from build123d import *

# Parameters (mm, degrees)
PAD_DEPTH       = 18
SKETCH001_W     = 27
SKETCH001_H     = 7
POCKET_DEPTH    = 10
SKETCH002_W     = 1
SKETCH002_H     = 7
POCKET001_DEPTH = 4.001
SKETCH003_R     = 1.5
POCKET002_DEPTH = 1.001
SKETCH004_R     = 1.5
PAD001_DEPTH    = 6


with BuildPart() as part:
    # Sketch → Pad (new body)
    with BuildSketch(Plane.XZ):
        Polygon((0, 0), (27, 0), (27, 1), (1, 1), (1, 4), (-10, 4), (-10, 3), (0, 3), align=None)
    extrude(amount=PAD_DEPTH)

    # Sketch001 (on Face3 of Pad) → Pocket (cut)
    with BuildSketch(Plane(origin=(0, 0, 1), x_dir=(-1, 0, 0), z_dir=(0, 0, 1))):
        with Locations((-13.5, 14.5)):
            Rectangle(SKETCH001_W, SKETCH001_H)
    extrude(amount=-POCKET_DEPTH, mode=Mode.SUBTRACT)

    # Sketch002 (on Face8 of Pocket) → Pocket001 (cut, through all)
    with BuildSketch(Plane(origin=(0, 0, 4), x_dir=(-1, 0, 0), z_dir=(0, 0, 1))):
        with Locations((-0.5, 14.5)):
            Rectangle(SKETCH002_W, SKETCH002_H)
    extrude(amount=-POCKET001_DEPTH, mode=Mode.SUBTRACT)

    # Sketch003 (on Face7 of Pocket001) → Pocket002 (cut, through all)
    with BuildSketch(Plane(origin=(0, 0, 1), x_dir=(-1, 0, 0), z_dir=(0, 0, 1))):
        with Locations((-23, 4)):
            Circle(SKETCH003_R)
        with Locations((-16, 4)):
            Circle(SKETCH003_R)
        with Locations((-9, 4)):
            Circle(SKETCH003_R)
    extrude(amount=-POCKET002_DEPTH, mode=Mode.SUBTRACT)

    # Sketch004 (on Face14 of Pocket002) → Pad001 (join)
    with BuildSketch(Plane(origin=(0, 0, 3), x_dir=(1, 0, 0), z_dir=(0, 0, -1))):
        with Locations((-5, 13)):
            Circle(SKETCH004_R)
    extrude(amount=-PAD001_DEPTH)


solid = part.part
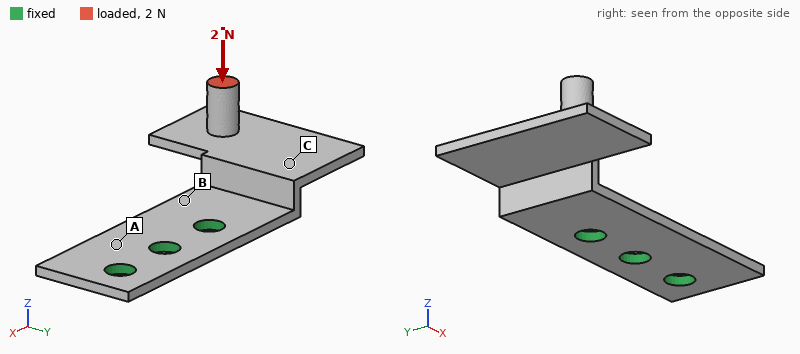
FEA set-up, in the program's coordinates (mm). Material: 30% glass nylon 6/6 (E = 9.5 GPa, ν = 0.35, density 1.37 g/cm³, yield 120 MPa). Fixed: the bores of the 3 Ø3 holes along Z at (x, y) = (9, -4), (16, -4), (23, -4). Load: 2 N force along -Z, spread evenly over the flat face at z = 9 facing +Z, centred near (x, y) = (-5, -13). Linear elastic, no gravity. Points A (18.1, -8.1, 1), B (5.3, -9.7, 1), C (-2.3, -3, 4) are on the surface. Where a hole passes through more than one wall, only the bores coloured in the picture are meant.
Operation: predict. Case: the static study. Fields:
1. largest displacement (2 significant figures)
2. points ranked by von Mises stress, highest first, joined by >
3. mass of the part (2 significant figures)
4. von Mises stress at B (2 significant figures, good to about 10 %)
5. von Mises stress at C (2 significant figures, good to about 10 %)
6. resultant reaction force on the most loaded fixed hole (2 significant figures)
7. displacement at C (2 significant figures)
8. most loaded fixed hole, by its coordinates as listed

0.49 mm
B > C > A
0.72 g
11 MPa
4.3 MPa
2.8 N
0.12 mm
(9, -4)
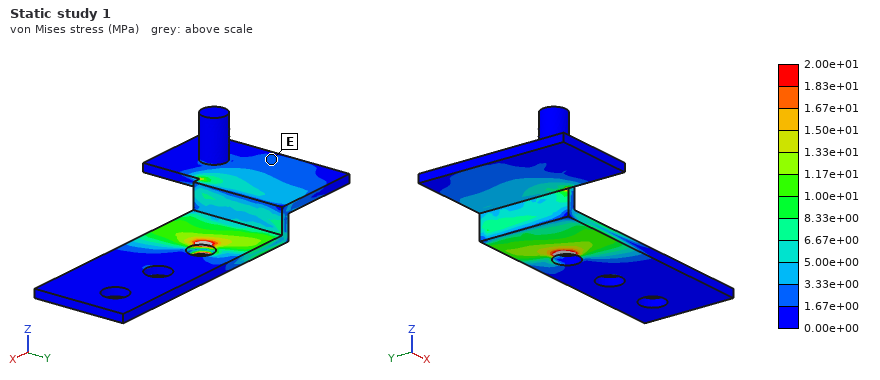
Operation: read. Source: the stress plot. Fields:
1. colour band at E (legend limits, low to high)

1.67e+00 to 3.33e+00 MPa
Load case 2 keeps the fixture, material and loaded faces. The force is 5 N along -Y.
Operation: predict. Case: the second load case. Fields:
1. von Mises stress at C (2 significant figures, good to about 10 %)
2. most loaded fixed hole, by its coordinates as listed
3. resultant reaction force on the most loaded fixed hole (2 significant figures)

3.5 MPa
(9, -4)
9.6 N
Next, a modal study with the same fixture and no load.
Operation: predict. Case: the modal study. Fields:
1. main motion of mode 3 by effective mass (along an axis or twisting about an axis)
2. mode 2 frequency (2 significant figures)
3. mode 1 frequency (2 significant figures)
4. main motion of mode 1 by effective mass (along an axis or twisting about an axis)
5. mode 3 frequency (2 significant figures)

along Y
1900 Hz
780 Hz
along Z
3100 Hz
